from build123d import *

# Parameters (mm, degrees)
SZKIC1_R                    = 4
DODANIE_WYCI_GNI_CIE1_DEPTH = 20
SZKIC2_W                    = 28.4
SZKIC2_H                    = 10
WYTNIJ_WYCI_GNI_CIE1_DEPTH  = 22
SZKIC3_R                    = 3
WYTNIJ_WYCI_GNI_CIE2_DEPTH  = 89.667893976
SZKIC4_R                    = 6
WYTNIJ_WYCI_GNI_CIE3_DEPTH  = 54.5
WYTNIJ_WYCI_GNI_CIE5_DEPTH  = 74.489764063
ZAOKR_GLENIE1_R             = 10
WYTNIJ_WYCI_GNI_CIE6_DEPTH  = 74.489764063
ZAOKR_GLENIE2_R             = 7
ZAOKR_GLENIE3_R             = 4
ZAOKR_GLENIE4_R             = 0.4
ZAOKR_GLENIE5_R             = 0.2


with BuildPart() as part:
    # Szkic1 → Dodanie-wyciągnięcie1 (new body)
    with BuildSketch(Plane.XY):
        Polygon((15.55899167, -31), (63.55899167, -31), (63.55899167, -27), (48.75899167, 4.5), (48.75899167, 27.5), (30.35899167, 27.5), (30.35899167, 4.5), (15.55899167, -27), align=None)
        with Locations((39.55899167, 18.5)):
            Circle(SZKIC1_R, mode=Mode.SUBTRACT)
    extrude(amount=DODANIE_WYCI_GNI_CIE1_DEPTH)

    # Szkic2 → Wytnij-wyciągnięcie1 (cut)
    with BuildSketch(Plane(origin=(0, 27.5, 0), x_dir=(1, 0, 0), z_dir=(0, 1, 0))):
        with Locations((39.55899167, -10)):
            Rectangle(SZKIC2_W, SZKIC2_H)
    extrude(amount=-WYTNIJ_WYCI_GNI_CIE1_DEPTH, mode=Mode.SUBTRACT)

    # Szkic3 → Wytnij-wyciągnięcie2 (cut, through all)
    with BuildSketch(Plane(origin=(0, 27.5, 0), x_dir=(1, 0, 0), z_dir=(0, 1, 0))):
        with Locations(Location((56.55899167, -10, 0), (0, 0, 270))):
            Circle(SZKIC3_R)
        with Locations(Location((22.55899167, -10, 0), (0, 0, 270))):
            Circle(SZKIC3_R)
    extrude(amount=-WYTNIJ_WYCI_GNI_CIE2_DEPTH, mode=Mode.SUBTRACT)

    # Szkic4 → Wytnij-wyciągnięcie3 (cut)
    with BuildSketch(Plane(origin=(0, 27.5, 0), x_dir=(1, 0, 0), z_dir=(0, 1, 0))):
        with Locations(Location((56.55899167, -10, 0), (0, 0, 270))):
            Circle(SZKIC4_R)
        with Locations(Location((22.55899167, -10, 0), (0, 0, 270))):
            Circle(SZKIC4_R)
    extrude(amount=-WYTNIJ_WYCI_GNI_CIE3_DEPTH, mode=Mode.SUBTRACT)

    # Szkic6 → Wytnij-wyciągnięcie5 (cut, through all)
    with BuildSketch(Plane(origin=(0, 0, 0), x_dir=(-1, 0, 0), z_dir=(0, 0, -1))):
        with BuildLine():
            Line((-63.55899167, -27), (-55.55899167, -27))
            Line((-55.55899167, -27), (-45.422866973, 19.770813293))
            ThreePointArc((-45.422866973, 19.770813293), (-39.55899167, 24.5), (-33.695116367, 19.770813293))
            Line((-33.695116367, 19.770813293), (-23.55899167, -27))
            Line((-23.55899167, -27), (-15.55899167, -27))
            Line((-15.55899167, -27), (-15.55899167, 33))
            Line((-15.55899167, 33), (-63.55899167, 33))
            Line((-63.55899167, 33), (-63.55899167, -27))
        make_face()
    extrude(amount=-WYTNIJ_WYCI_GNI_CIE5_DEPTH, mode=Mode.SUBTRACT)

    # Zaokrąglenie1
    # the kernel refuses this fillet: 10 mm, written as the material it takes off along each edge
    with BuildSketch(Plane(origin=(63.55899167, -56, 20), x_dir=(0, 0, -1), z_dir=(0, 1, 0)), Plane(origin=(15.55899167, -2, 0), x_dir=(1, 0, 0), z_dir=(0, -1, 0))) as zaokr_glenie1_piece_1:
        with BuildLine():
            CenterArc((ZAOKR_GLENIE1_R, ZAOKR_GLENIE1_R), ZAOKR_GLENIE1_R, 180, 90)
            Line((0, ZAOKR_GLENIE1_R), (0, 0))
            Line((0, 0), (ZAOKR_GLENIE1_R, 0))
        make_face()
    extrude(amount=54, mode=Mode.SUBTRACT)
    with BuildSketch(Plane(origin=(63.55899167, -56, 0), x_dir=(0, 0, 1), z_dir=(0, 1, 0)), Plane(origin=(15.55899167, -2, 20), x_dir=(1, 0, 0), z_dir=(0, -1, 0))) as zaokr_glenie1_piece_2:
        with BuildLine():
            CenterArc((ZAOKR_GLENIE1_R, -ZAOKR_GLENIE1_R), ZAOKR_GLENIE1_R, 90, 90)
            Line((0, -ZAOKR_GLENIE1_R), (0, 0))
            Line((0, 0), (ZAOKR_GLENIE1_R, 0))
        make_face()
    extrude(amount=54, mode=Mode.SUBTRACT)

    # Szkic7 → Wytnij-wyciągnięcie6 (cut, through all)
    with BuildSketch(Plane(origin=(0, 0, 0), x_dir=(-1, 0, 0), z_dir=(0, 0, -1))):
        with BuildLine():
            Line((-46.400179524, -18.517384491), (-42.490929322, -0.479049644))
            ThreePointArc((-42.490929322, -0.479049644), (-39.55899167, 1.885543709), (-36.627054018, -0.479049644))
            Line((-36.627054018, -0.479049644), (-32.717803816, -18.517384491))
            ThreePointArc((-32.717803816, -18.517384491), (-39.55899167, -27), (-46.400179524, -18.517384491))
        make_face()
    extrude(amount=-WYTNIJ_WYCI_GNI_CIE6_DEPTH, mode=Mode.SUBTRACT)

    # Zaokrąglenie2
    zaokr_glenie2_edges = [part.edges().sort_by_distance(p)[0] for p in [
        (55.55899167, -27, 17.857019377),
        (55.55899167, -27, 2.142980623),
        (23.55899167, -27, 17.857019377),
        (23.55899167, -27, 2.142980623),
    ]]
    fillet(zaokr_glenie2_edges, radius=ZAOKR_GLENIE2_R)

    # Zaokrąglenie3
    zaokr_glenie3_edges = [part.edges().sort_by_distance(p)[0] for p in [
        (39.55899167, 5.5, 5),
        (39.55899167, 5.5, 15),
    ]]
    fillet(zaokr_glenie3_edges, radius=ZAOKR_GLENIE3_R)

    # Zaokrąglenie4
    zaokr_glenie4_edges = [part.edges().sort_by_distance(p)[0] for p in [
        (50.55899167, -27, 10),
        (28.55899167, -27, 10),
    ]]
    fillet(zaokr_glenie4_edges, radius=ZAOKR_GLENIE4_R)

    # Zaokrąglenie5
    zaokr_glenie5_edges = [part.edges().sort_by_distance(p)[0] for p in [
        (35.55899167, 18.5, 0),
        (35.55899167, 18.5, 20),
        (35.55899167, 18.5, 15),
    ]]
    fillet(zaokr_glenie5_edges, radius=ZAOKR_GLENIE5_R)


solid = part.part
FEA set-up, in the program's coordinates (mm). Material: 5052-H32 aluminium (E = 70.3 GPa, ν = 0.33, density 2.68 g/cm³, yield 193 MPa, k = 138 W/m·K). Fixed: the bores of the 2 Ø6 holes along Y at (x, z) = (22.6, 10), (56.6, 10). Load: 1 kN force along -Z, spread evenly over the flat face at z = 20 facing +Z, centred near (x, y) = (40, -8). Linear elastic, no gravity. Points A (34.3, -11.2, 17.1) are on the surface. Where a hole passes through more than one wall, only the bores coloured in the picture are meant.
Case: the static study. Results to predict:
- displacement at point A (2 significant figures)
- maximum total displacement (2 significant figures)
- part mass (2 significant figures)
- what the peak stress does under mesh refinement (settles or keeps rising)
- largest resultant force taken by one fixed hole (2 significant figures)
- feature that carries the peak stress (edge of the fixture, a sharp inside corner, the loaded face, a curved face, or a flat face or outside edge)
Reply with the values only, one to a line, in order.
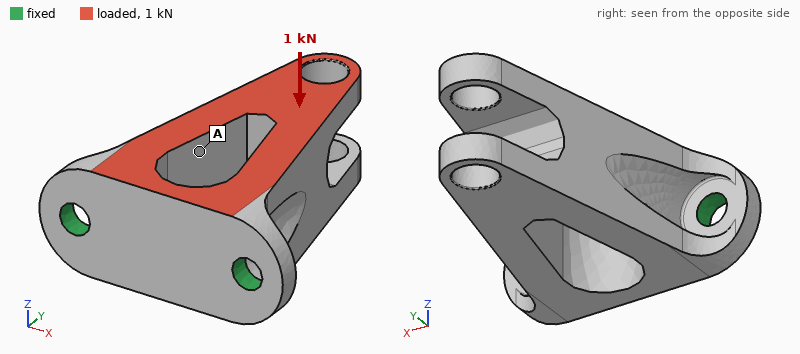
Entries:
0.050 mm
0.16 mm
41 g
keeps rising
500 N
edge of the fixture
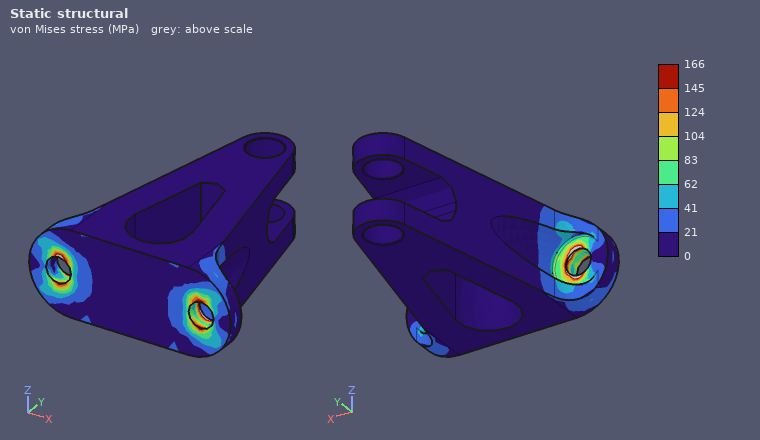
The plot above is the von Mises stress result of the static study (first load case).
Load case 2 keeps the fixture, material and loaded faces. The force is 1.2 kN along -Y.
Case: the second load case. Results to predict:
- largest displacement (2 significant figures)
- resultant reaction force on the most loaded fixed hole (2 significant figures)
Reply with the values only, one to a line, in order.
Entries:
90 µm
620 N
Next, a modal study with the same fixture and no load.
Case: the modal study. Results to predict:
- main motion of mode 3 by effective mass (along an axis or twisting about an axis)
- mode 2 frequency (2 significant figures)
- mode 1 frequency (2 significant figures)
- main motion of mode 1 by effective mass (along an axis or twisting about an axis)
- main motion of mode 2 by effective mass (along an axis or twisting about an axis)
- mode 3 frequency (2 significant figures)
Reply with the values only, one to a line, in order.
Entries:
twisting about Y
6700 Hz
3000 Hz
along Z
along X
11 kHz
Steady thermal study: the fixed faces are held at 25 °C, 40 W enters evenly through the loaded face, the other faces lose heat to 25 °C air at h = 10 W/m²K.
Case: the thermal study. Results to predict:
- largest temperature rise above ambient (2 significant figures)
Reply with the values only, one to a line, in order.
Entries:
40 K
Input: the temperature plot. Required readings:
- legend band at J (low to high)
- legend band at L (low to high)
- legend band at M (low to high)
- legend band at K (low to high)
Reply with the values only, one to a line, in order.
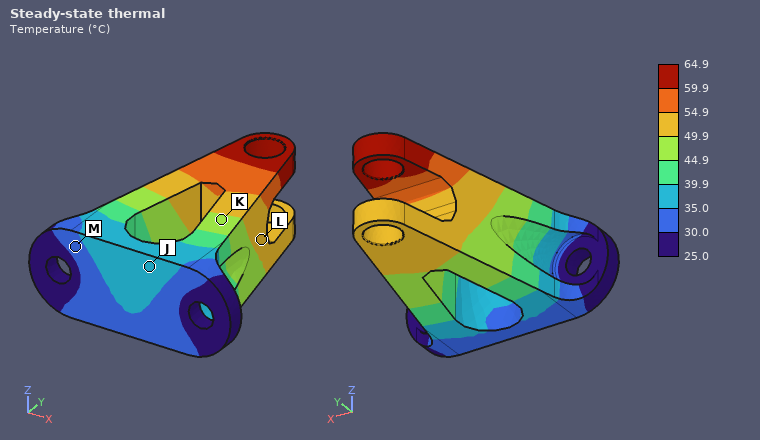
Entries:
35.0 to 39.9 °C
49.9 to 54.9 °C
30.0 to 35.0 °C
44.9 to 49.9 °C
